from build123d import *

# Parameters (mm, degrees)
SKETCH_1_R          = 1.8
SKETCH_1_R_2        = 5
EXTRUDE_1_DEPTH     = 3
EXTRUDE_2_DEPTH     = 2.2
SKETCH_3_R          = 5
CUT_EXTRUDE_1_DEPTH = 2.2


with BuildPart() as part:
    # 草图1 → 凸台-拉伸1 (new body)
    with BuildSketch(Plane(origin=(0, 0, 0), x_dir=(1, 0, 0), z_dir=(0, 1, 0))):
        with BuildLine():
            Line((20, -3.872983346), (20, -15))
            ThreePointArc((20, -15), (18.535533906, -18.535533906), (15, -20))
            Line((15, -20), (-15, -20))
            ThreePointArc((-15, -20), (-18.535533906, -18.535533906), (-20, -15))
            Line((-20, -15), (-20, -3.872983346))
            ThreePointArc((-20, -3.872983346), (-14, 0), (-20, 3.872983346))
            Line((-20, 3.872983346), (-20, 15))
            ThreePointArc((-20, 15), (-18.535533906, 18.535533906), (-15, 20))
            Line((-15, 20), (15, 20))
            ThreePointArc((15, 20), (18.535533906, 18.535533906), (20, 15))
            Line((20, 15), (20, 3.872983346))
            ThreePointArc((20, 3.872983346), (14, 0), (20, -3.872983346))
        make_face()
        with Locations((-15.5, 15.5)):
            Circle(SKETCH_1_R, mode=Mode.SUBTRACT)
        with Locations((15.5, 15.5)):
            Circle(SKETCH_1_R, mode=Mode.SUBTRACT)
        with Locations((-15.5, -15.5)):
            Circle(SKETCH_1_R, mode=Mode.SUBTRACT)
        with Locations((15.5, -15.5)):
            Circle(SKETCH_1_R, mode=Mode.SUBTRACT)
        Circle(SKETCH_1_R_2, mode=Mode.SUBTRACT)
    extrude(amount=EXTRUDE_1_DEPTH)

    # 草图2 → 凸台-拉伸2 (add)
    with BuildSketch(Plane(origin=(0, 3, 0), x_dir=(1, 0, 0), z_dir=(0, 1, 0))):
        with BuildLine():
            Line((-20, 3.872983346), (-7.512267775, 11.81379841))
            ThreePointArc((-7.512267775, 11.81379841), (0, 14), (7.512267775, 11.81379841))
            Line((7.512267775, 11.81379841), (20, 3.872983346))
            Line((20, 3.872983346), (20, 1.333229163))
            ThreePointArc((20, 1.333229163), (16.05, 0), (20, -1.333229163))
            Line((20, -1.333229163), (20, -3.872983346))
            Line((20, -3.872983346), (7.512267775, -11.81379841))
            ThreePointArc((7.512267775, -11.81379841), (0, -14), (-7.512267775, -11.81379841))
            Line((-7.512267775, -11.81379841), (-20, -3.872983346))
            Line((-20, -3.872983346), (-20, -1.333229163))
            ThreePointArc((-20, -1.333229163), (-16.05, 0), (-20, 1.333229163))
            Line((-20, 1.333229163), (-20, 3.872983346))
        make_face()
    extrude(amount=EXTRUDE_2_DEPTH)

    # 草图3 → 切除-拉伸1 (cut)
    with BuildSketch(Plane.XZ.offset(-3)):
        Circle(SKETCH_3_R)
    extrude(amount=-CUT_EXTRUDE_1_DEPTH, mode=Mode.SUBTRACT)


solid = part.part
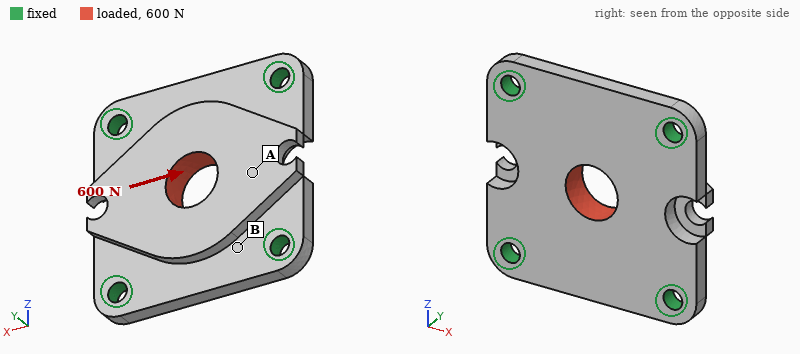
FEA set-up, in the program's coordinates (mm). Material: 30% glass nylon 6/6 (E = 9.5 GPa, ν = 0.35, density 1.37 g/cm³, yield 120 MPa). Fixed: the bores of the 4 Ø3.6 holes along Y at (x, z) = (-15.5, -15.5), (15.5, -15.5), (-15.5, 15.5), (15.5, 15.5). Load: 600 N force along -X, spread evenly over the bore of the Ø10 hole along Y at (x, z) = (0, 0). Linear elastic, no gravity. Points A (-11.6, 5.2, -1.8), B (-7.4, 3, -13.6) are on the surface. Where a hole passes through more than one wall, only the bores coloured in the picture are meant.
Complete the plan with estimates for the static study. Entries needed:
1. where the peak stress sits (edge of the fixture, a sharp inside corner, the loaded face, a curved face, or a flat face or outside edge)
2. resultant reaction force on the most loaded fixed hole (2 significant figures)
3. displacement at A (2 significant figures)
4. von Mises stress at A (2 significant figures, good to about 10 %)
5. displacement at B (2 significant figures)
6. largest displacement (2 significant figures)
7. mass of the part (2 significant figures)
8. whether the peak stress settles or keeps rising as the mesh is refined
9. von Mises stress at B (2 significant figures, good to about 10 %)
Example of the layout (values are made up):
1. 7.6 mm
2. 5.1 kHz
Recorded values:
1. edge of the fixture
2. 170 N
3. 10 µm
4. 1.9 MPa
5. 3.9 µm
6. 12 µm
7. 7.7 g
8. keeps rising
9. 5.3 MPa
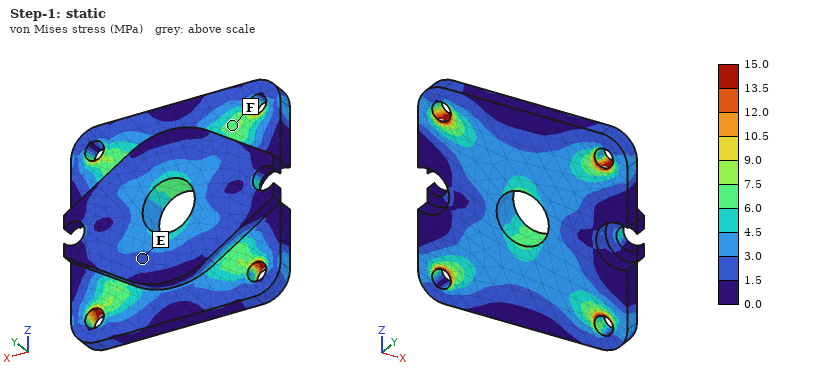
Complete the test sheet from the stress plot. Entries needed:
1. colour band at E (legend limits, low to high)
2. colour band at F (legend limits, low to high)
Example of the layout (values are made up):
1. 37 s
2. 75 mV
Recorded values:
1. 1.5 to 3.0 MPa
2. 6.0 to 7.5 MPa
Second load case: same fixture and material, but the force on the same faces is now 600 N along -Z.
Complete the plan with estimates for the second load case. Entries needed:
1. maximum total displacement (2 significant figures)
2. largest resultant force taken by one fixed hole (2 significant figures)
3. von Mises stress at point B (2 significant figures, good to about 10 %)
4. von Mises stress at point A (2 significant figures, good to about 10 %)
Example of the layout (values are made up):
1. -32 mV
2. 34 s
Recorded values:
1. 12 µm
2. 170 N
3. 4.6 MPa
4. 2.1 MPa
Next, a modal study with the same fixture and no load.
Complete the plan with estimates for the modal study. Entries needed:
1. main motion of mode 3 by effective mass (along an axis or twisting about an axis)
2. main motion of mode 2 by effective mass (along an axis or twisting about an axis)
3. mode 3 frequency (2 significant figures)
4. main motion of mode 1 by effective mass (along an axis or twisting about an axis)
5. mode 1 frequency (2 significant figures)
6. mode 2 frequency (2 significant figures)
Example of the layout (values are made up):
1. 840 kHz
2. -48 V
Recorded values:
1. twisting about Z
2. twisting about X
3. 11 kHz
4. along Y
5. 7000 Hz
6. 10 kHz
